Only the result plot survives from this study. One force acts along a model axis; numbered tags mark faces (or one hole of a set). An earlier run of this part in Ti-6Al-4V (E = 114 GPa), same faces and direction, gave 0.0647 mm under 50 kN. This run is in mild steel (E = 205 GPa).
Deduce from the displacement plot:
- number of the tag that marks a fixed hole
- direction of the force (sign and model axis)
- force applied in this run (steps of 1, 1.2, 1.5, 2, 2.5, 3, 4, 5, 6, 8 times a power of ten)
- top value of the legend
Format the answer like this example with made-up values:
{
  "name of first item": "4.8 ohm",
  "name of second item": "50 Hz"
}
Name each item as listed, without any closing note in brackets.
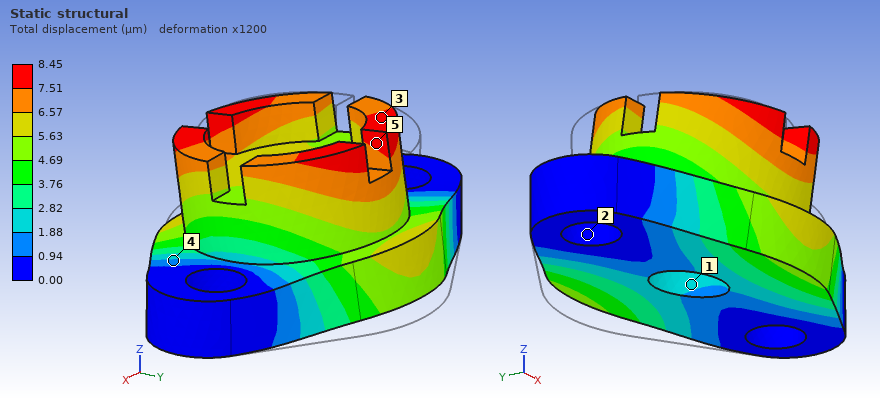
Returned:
{
  "number of the tag that marks a fixed hole": "2",
  "direction of the force": "-Y",
  "force applied in this run": "12 kN",
  "top value of the legend": "8.45 µm"
}
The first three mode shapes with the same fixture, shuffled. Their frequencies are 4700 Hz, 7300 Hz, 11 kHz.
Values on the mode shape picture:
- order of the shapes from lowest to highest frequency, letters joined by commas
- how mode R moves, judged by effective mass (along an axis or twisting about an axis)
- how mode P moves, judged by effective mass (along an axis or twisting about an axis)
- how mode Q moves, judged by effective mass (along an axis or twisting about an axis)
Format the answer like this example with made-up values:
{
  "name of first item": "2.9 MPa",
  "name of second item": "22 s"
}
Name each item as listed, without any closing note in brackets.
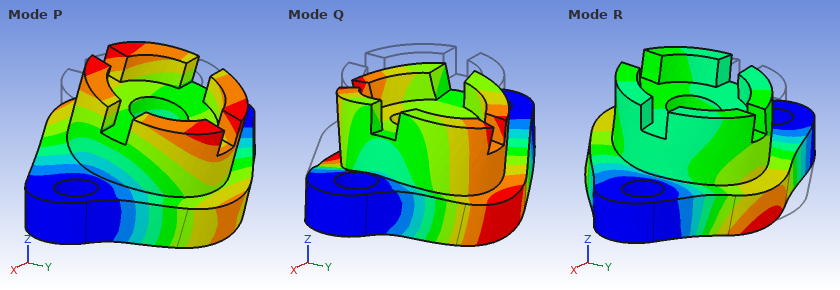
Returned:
{
  "order of the shapes from lowest to highest frequency, letters joined by commas": "P, Q, R",
  "how mode R moves, judged by effective mass": "along Y",
  "how mode P moves, judged by effective mass": "along Y",
  "how mode Q moves, judged by effective mass": "along Z"
}
